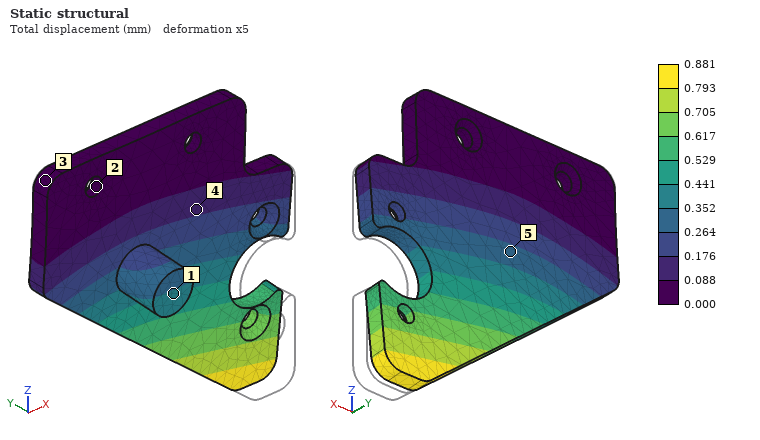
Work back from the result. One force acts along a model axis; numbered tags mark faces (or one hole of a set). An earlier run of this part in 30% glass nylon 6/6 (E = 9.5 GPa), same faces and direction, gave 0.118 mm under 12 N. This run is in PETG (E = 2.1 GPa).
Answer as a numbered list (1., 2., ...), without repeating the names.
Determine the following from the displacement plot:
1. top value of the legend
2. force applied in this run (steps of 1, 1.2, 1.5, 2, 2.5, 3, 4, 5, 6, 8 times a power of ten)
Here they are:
1. 0.881 mm
2. 20 N
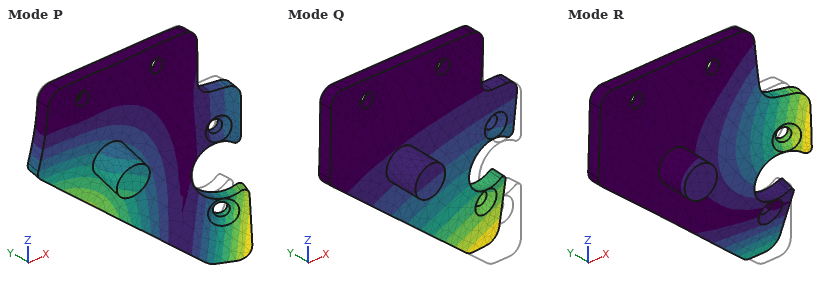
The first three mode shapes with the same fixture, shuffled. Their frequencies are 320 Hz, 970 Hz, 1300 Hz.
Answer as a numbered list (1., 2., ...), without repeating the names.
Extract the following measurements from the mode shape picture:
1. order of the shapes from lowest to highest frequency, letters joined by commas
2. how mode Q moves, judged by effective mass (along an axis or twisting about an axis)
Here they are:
1. Q, P, R
2. along Y
